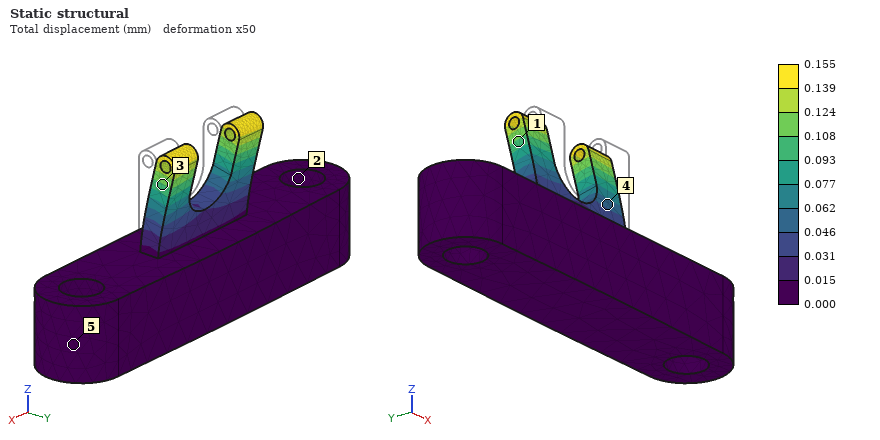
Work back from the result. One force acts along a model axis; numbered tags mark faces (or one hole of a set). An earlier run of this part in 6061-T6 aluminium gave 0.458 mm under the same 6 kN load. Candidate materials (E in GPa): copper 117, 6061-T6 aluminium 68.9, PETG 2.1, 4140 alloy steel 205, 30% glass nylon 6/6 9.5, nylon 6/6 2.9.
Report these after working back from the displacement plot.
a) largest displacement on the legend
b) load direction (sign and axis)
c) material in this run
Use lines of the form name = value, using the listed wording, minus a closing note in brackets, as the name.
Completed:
largest displacement on the legend = 0.155 mm
load direction = +Y
material in this run = 4140 alloy steel
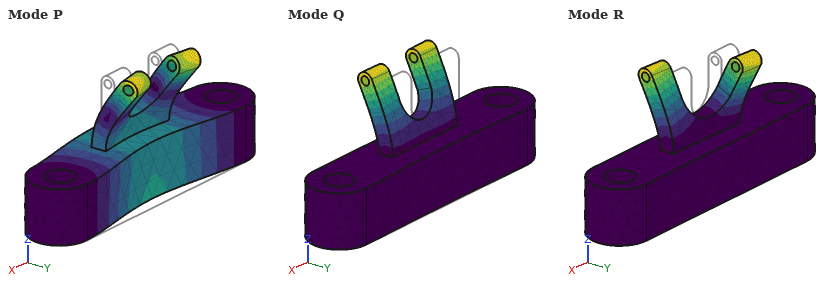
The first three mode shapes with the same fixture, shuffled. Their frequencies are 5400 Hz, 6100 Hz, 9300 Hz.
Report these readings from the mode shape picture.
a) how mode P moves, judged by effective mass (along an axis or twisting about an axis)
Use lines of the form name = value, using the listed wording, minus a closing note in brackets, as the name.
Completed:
how mode P moves, judged by effective mass = along Y
